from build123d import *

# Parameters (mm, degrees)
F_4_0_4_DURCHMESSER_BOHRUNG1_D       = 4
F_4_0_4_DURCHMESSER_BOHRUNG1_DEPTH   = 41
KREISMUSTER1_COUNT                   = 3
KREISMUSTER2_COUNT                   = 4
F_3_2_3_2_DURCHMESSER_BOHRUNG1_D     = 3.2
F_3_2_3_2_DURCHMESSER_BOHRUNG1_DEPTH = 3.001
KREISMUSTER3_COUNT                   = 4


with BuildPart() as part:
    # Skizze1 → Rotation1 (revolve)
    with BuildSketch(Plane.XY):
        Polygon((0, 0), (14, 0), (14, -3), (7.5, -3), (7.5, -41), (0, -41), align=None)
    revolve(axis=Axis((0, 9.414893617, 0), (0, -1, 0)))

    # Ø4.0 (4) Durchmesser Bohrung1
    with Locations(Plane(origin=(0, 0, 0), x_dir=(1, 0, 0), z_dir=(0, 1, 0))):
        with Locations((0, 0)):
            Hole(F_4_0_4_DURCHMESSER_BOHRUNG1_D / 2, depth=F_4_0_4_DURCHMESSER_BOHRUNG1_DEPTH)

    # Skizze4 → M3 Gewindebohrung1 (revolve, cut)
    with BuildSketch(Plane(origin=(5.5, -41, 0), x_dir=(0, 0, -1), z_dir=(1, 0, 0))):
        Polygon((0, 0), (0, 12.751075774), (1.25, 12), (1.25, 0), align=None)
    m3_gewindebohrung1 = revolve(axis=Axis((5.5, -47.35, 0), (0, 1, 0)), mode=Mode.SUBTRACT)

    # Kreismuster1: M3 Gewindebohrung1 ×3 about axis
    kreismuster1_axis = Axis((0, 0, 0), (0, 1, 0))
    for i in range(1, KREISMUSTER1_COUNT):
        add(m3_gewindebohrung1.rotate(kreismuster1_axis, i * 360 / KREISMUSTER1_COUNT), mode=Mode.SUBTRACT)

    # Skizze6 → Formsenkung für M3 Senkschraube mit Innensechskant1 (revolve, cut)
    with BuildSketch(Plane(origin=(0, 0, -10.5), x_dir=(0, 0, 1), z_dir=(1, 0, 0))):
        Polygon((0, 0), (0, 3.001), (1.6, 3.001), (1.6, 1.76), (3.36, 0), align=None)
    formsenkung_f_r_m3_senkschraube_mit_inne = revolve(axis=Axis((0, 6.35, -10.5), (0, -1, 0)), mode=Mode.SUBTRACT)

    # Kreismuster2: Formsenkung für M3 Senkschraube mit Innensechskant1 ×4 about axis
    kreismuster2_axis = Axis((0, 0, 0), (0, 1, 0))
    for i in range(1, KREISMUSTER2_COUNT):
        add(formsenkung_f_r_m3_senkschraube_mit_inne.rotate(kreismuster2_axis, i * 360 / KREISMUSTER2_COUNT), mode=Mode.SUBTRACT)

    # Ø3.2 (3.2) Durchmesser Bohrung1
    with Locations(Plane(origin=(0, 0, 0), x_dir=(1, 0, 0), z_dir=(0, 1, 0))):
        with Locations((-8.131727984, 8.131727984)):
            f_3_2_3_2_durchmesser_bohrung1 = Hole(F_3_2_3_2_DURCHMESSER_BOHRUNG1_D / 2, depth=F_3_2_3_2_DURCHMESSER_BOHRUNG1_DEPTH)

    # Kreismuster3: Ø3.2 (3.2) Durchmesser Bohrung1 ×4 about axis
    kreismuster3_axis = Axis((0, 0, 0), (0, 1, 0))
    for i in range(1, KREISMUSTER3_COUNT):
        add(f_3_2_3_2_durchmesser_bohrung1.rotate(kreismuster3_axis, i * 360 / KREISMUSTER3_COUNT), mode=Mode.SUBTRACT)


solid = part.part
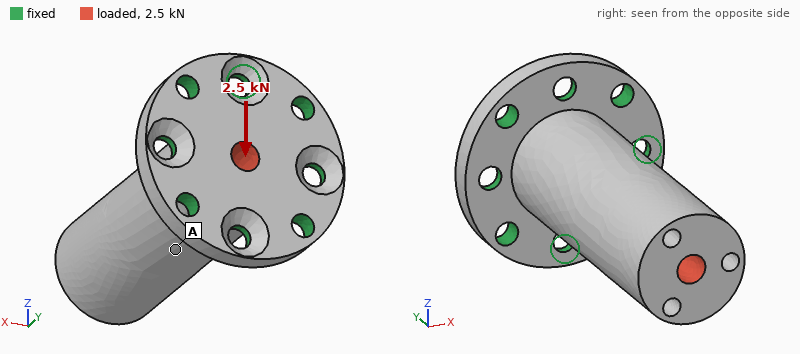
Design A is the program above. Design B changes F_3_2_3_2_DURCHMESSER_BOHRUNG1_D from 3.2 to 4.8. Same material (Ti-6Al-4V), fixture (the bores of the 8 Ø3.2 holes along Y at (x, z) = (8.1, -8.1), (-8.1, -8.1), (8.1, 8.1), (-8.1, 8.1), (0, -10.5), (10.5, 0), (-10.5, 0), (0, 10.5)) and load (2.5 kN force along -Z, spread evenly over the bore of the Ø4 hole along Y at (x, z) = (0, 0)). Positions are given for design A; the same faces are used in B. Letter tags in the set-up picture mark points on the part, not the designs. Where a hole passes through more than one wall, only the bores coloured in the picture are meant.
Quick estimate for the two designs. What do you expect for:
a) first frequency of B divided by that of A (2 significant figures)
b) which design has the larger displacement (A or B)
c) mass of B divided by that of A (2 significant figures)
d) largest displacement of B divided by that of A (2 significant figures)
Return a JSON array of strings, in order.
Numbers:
["1.0", "A", "0.98", "0.92"]
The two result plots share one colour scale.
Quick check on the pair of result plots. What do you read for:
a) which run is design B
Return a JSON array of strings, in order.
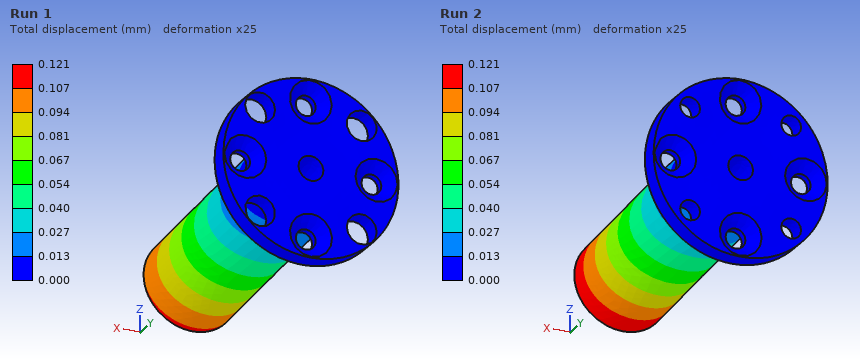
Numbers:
["Run 1"]
